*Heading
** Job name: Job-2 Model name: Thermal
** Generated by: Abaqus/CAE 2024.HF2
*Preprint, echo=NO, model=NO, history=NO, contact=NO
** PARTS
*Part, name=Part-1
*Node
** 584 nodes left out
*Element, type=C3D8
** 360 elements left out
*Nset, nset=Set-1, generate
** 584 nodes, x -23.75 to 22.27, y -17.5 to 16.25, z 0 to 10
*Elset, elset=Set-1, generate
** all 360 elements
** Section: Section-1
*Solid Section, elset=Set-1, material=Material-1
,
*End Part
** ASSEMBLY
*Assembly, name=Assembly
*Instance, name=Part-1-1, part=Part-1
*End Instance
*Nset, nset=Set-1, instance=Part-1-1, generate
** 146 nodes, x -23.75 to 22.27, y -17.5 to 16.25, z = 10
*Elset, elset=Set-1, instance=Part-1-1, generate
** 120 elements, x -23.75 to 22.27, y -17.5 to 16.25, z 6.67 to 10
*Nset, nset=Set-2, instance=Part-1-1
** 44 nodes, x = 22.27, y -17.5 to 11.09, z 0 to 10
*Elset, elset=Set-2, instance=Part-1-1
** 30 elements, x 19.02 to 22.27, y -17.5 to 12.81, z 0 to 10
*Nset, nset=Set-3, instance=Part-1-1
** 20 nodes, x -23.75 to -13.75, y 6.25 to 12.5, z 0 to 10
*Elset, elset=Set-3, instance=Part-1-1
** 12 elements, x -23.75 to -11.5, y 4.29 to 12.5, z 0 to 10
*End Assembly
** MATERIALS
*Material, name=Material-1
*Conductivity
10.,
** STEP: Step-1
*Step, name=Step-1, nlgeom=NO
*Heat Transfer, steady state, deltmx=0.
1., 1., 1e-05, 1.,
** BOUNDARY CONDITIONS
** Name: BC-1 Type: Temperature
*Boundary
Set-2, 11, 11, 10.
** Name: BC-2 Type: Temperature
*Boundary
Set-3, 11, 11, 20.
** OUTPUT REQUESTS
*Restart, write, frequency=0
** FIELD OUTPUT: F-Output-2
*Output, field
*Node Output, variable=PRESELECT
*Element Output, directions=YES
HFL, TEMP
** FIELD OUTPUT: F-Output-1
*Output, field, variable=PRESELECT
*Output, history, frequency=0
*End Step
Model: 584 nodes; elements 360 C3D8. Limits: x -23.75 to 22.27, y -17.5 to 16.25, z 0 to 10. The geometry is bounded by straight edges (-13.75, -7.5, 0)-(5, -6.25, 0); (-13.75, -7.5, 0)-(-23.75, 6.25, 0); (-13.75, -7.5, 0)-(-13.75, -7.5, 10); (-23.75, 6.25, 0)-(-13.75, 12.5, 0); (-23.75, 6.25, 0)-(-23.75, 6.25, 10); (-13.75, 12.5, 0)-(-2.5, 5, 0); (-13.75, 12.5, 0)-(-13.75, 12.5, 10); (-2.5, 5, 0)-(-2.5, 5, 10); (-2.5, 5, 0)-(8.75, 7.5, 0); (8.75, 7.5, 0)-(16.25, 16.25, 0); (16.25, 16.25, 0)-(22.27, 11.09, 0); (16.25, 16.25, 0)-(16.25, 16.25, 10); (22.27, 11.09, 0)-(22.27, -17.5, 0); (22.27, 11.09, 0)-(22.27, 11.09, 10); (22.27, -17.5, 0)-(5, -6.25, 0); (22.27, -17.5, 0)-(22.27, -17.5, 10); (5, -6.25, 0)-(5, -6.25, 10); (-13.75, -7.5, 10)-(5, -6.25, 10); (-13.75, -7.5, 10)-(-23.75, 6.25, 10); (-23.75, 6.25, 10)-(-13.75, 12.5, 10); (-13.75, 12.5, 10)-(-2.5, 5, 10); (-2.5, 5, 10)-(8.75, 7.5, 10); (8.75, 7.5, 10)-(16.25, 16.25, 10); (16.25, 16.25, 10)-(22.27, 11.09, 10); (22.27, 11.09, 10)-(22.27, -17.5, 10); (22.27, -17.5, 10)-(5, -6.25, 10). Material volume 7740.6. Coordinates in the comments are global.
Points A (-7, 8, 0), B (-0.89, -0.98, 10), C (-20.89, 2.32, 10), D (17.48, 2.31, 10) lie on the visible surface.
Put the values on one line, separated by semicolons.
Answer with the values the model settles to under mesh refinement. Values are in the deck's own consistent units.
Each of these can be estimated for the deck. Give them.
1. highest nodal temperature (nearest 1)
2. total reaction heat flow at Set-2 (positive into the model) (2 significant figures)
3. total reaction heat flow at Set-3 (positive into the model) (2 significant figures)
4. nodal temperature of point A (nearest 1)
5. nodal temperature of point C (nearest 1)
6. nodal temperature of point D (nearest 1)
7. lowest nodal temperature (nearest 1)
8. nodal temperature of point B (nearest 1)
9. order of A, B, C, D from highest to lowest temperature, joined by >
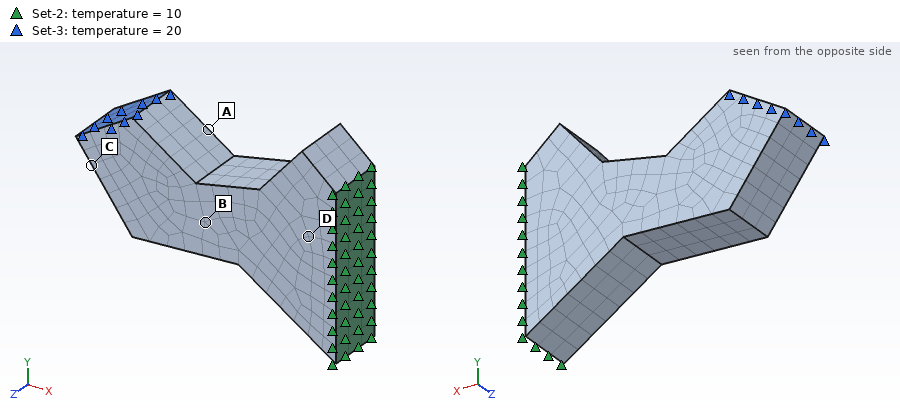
20; -340; 340; 17; 19; 11; 10; 15; C > A > B > D
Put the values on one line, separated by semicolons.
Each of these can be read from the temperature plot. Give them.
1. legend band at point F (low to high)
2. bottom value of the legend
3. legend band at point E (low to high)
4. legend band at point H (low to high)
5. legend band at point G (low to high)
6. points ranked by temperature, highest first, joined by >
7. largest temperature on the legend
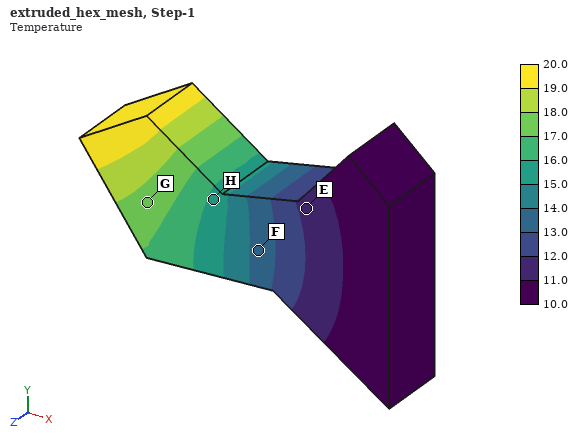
13.0 to 14.0; 10.0; 11.0 to 12.0; 15.0 to 16.0; 17.0 to 18.0; G > H > F > E; 20.0
